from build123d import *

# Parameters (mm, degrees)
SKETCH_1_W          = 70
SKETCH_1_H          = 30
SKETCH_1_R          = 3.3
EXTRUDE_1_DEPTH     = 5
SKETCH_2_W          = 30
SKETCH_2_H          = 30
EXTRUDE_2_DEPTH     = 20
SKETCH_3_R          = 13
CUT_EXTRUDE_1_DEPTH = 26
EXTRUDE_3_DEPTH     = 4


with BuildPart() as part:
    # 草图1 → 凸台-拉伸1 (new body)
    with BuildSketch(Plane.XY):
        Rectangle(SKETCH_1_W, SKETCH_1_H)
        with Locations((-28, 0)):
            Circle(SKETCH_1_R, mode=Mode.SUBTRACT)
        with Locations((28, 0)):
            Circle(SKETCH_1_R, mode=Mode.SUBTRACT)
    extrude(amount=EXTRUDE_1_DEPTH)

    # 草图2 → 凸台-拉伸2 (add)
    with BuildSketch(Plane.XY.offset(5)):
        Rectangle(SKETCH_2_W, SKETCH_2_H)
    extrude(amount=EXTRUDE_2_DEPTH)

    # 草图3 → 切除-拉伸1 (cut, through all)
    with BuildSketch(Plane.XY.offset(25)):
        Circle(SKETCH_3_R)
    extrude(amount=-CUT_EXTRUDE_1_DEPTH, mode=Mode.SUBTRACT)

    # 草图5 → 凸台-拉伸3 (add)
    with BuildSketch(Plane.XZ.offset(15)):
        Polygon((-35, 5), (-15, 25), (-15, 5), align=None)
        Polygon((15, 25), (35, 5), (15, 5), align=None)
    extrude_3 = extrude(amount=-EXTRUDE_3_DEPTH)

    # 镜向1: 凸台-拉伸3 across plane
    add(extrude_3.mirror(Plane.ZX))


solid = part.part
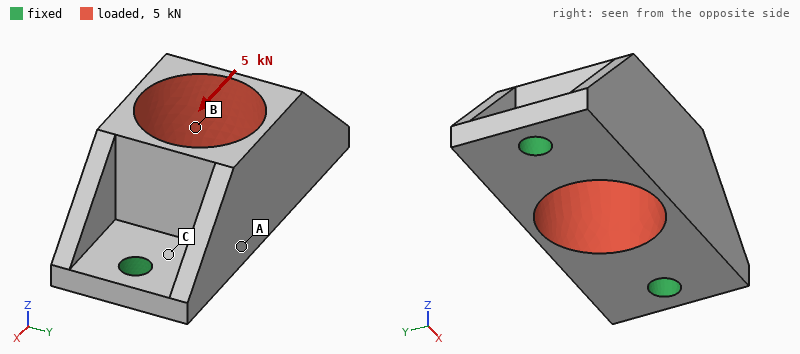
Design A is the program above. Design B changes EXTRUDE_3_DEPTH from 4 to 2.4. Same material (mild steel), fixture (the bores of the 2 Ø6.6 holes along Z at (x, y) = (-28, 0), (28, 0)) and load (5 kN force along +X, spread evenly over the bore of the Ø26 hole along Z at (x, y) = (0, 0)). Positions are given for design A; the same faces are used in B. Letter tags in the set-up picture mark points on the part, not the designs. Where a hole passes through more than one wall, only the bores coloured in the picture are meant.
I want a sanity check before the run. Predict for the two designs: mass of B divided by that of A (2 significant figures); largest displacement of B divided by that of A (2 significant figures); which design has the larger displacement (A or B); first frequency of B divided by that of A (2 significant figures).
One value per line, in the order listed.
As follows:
0.93
1.2
B
1.0
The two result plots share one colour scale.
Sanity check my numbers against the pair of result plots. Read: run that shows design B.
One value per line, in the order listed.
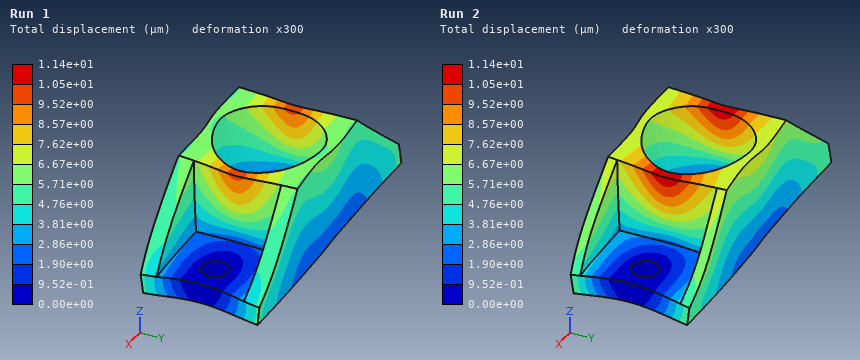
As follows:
Run 2
